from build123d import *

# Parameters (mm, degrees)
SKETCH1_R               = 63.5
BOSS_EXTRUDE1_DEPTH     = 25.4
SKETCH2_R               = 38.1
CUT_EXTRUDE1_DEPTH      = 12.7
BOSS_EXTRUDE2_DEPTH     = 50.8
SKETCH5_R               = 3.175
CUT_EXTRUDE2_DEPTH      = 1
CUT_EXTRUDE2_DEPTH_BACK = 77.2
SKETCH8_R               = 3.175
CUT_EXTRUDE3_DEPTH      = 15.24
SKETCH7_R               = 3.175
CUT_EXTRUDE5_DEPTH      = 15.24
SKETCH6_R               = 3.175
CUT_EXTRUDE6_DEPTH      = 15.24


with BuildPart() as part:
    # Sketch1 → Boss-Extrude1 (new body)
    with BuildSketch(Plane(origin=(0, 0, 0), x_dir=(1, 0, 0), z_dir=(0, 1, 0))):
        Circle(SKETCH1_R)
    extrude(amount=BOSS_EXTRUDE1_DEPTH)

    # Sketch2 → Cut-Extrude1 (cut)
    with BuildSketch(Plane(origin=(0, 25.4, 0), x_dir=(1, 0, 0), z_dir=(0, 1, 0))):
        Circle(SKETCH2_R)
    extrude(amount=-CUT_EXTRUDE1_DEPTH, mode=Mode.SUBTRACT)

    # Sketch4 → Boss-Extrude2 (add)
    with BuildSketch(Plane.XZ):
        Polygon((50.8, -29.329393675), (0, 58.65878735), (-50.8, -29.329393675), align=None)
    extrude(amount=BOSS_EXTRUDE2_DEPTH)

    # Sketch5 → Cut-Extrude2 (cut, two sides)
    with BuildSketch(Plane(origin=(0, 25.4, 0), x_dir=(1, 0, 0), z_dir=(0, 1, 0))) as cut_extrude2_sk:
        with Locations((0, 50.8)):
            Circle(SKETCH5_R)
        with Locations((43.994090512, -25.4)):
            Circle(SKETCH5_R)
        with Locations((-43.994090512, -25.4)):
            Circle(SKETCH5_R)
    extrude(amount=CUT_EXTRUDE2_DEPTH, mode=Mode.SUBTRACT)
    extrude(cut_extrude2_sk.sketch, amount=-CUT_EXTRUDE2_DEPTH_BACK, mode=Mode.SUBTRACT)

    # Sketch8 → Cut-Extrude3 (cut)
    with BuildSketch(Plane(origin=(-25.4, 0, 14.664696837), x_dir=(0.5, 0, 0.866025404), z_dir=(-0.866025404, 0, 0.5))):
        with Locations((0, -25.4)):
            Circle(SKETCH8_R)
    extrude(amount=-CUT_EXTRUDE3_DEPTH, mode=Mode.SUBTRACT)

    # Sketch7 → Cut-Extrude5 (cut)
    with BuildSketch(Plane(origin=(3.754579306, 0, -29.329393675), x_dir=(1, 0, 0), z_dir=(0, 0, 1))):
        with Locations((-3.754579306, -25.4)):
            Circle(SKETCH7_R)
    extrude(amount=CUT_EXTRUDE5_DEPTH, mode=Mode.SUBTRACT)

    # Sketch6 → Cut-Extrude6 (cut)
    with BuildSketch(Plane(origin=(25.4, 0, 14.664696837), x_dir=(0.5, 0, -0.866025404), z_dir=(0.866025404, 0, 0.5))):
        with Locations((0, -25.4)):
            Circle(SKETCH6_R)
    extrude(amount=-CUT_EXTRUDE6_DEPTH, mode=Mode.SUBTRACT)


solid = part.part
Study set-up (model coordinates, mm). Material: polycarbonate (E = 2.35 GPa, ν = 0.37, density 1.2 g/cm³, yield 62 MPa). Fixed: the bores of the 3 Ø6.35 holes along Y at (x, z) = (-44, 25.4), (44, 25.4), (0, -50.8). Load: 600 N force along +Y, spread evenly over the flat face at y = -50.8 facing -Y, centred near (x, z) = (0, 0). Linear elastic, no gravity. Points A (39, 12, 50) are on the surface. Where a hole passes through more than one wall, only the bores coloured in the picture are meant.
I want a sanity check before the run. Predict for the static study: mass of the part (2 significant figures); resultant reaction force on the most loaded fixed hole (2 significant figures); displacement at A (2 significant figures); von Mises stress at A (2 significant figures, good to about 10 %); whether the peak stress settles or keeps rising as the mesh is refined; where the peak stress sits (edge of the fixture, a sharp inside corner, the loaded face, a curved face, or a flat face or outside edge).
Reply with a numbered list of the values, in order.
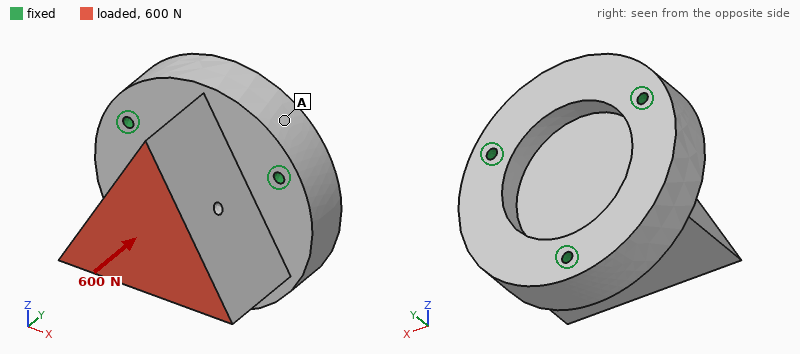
1. 580 g
2. 210 N
3. 3.9 µm
4. 0.16 MPa
5. keeps rising
6. edge of the fixture
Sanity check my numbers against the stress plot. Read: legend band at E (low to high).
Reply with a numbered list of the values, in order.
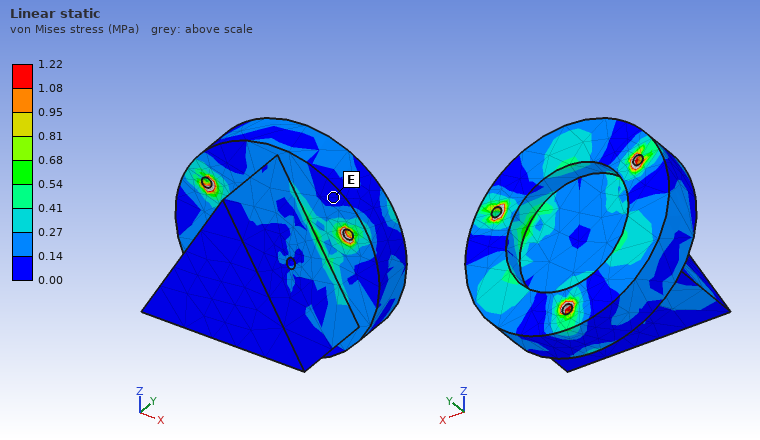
1. 0.00 to 0.14 MPa
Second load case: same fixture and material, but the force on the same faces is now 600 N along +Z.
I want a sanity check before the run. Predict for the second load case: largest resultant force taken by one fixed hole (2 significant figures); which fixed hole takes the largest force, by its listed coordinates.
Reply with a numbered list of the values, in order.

1. 520 N
2. (0, -50.8)
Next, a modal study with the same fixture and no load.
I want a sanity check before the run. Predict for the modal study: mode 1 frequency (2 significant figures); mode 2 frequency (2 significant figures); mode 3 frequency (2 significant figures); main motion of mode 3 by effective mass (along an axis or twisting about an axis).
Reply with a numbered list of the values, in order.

1. 1200 Hz
2. 1200 Hz
3. 1600 Hz
4. along Y
